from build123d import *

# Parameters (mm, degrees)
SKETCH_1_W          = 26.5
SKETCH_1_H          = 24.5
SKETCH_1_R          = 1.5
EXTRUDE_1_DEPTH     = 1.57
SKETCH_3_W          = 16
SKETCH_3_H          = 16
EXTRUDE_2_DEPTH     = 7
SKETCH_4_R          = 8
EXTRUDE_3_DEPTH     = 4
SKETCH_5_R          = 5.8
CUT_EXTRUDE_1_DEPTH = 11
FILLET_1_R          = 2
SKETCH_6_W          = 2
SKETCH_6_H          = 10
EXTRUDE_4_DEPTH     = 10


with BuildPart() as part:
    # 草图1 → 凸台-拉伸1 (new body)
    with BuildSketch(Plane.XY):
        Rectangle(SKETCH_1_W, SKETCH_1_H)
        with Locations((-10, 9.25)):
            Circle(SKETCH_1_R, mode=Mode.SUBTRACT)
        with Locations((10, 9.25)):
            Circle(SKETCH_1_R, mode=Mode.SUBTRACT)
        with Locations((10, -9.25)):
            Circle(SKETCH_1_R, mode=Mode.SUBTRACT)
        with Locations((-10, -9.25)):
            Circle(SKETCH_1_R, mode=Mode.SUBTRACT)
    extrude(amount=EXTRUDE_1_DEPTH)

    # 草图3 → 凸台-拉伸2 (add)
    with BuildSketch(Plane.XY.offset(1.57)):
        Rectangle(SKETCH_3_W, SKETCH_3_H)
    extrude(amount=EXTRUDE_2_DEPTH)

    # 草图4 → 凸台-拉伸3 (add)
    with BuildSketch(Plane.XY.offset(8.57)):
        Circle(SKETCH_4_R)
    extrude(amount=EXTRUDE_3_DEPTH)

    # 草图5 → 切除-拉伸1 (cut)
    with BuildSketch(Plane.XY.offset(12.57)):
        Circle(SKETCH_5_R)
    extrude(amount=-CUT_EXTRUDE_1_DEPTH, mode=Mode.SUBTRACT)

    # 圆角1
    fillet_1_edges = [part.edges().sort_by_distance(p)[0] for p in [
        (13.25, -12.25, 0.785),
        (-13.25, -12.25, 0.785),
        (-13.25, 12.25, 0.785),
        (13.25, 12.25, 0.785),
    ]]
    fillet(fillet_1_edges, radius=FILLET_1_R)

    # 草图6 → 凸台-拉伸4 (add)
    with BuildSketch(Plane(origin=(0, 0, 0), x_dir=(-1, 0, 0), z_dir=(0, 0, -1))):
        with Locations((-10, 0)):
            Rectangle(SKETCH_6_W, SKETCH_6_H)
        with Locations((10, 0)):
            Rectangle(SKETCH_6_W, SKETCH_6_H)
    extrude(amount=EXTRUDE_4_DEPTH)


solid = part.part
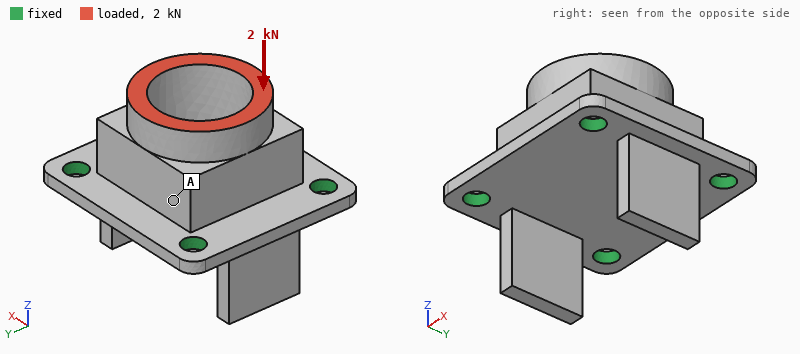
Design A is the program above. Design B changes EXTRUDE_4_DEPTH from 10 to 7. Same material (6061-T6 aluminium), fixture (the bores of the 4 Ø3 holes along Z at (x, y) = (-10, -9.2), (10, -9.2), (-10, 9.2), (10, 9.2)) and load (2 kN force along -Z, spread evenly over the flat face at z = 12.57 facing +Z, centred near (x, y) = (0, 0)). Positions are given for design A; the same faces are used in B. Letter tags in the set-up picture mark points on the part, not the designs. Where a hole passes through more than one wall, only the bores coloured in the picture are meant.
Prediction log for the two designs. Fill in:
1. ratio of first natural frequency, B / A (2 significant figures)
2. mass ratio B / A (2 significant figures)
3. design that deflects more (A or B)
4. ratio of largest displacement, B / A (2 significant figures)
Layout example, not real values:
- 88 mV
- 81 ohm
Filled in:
- 1.7
- 0.96
- A
- 0.78
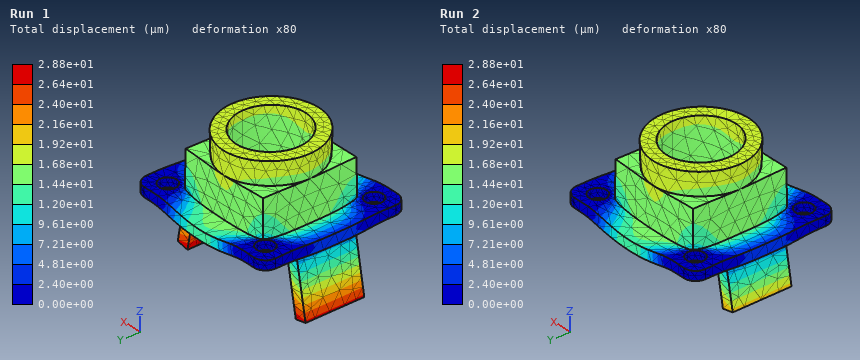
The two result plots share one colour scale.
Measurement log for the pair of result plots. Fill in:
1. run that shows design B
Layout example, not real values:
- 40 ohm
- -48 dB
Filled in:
- Run 2
